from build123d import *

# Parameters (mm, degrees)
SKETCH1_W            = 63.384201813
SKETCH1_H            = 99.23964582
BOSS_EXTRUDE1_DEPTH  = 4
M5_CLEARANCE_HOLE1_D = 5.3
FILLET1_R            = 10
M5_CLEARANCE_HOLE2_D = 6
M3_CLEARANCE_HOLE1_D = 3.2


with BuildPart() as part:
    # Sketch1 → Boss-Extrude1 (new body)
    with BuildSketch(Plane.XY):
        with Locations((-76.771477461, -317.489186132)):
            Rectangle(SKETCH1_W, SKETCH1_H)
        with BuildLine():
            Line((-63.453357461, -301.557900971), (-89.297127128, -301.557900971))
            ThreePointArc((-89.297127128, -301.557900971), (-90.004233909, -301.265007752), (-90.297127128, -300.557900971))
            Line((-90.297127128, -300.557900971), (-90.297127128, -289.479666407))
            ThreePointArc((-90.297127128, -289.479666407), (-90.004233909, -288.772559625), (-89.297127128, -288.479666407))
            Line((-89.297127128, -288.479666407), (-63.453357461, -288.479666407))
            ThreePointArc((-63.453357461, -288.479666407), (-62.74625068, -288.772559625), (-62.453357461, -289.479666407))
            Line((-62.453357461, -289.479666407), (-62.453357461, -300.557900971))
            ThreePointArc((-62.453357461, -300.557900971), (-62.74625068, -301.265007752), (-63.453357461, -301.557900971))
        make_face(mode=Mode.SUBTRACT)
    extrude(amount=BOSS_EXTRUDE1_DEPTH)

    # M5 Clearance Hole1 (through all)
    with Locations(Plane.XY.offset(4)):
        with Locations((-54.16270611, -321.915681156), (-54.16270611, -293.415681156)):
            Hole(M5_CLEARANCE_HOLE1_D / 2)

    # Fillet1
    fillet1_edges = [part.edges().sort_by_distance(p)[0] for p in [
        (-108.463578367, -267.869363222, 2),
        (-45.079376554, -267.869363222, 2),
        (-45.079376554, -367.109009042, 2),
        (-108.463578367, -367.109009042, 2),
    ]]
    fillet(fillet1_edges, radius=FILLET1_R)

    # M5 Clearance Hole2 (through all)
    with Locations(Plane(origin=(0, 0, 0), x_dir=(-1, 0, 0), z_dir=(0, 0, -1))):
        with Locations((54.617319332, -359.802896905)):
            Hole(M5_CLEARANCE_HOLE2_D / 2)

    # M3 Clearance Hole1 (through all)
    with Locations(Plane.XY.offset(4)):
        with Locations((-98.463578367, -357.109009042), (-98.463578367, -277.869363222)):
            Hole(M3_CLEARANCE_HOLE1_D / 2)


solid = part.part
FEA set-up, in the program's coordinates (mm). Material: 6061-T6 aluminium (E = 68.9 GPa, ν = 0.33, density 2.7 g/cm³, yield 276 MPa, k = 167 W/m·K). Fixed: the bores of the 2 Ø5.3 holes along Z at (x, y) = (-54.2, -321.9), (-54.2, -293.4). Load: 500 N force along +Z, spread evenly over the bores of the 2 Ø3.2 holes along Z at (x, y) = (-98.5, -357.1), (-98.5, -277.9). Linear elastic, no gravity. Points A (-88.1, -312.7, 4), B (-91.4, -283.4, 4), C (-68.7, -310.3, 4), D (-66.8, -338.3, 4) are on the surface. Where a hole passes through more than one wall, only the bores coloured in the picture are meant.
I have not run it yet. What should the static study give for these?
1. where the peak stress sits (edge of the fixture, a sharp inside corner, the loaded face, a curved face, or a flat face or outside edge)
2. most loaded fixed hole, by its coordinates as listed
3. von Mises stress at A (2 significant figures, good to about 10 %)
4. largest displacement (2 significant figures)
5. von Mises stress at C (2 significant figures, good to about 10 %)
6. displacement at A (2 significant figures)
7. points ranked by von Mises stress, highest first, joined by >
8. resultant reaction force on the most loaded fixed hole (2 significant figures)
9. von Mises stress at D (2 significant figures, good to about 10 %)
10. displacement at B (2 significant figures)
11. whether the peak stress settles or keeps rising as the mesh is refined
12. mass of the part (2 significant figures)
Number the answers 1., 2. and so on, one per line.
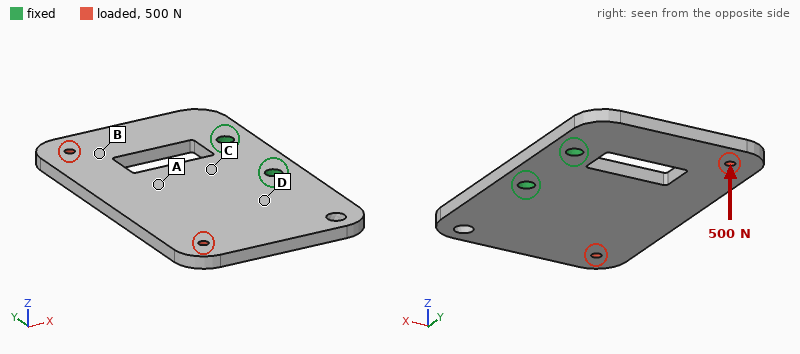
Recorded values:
1. edge of the fixture
2. (-54.2, -321.9)
3. 36 MPa
4. 1.1 mm
5. 85 MPa
6. 0.37 mm
7. C > D > A > B
8. 440 N
9. 57 MPa
10. 0.50 mm
11. keeps rising
12. 62 g
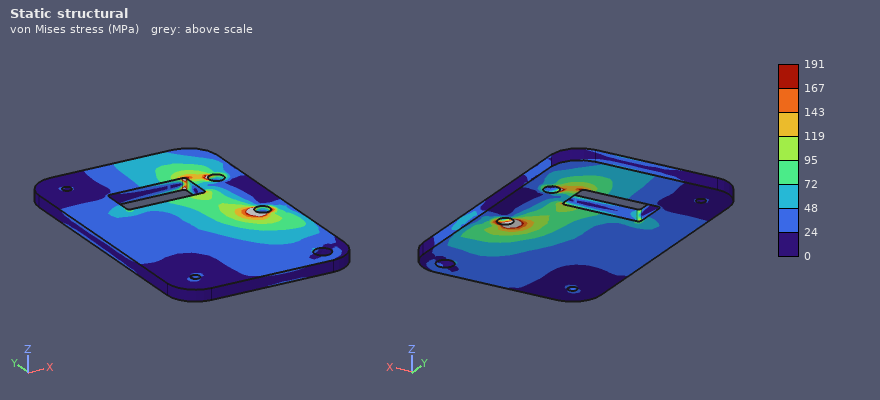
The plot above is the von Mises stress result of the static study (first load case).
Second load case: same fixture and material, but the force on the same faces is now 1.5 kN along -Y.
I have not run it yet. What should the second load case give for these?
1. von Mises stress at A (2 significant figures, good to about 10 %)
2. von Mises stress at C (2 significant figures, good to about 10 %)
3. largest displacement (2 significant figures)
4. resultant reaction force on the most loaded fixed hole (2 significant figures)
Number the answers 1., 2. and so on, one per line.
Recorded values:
1. 17 MPa
2. 31 MPa
3. 84 µm
4. 2.1 kN
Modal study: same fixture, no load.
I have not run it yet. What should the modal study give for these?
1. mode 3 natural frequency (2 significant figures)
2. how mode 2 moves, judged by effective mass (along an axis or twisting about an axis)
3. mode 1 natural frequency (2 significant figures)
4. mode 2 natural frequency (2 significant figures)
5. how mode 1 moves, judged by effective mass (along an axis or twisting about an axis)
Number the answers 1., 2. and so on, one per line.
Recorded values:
1. 2200 Hz
2. twisting about X
3. 860 Hz
4. 1200 Hz
5. along Z
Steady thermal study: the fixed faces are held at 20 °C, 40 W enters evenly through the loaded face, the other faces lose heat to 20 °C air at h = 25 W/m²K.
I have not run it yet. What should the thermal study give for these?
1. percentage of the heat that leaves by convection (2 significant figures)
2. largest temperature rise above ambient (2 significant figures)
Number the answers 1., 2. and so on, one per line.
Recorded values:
1. 18 %
2. 50 K
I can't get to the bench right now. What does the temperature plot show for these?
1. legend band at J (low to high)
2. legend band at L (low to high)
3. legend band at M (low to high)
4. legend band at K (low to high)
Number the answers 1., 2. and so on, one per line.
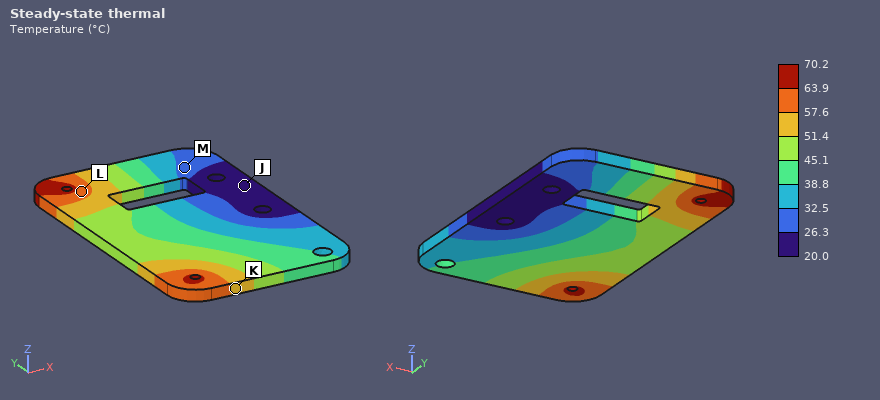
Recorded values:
1. 20.0 to 26.3 °C
2. 57.6 to 63.9 °C
3. 26.3 to 32.5 °C
4. 51.4 to 57.6 °C
